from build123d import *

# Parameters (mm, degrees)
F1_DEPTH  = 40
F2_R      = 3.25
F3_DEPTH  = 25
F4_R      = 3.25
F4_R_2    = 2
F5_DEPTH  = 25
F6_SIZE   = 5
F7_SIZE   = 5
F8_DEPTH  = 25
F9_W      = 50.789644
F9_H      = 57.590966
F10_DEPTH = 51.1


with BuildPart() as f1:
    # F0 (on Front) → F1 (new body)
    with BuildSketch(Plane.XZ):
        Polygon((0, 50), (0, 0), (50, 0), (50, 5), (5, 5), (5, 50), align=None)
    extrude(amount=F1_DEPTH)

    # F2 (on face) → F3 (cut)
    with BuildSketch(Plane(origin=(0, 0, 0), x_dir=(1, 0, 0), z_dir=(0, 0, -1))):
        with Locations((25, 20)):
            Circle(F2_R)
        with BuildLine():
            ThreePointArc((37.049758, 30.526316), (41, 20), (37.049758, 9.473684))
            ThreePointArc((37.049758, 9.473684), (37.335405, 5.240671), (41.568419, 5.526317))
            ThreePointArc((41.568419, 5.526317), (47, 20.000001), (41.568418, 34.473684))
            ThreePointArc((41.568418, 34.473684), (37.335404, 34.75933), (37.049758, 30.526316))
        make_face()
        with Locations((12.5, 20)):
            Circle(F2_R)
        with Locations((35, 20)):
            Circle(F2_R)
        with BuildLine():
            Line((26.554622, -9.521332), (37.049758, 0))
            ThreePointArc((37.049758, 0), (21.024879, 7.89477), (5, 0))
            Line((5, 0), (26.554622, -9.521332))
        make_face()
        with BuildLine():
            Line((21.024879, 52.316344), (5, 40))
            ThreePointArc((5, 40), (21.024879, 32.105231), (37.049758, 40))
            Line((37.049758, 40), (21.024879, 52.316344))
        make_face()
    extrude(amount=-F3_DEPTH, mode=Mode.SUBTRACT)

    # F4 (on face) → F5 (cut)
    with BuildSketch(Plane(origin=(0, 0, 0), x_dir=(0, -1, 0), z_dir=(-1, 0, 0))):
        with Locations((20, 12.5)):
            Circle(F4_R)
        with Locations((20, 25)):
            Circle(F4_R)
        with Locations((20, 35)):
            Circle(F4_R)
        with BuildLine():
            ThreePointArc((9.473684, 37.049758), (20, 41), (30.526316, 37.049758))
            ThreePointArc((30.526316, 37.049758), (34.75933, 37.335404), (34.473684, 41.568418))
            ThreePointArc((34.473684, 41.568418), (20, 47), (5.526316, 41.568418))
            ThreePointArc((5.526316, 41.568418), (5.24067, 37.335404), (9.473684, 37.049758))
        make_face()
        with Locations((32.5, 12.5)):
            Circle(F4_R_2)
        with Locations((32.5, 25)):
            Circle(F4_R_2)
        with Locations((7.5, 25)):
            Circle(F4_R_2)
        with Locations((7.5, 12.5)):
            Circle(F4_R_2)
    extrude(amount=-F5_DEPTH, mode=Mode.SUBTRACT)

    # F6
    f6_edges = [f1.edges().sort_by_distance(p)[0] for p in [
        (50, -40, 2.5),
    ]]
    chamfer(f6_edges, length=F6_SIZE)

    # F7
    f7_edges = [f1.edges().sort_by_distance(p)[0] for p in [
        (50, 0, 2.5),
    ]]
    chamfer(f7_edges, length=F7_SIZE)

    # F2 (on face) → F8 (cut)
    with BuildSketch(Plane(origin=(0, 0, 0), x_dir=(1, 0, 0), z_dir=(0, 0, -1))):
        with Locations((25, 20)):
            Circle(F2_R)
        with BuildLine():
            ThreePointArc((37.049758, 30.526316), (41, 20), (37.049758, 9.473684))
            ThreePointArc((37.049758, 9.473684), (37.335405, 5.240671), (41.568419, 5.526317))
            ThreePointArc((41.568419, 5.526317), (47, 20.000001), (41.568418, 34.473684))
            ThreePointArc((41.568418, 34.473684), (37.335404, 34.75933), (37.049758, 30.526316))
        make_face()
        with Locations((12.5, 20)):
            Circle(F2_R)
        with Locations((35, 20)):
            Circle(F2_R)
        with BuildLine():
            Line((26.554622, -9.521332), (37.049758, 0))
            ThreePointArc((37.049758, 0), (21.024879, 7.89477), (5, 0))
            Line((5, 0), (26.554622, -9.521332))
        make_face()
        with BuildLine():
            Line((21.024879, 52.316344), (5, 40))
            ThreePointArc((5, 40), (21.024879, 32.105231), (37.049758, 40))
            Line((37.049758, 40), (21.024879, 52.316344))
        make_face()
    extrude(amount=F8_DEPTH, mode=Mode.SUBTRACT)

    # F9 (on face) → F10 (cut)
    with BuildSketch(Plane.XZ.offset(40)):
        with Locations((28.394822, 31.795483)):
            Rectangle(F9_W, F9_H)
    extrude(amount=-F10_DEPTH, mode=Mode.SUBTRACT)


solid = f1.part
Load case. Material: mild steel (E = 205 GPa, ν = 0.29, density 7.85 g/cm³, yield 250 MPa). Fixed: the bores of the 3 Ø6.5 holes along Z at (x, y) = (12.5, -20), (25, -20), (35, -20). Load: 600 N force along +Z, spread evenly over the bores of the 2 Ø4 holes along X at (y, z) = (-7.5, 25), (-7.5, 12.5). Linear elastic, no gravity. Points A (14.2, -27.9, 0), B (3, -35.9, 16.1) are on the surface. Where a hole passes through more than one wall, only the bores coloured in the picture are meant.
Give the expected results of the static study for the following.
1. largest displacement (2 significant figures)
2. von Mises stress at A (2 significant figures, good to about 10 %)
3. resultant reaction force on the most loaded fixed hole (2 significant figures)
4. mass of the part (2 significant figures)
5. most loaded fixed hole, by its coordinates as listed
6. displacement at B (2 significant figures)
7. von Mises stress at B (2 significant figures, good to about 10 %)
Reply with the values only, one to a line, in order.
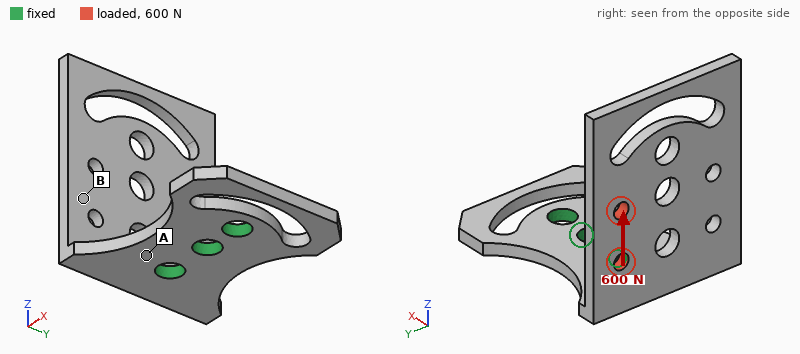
0.18 mm
52 MPa
690 N
68 g
(12.5, -20)
0.047 mm
22 MPa
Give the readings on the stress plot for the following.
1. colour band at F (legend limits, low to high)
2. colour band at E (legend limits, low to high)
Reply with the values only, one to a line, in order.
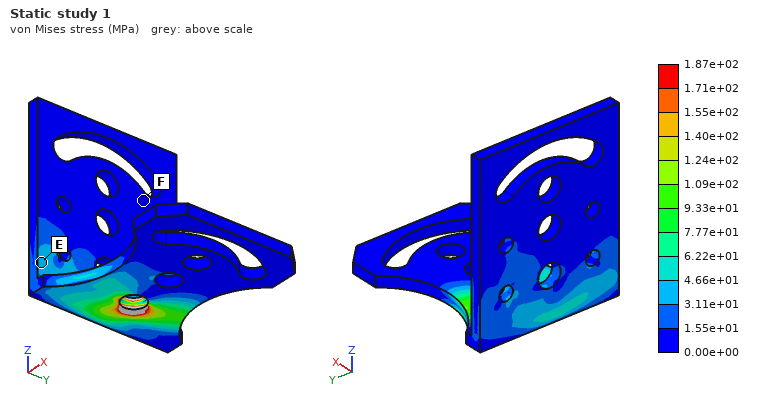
0.00e+00 to 1.55e+01 MPa
3.11e+01 to 4.66e+01 MPa
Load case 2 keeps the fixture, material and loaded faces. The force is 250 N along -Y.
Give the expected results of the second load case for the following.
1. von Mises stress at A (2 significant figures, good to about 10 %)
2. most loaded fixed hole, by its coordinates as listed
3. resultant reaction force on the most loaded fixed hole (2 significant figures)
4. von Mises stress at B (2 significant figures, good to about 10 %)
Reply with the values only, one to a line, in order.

44 MPa
(12.5, -20)
330 N
12 MPa
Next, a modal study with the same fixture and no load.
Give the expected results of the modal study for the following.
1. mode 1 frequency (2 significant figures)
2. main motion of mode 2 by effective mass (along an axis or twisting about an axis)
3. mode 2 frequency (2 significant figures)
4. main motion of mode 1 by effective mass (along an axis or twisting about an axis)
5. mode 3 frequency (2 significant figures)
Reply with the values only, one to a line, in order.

850 Hz
along Y
1500 Hz
along X
2600 Hz
